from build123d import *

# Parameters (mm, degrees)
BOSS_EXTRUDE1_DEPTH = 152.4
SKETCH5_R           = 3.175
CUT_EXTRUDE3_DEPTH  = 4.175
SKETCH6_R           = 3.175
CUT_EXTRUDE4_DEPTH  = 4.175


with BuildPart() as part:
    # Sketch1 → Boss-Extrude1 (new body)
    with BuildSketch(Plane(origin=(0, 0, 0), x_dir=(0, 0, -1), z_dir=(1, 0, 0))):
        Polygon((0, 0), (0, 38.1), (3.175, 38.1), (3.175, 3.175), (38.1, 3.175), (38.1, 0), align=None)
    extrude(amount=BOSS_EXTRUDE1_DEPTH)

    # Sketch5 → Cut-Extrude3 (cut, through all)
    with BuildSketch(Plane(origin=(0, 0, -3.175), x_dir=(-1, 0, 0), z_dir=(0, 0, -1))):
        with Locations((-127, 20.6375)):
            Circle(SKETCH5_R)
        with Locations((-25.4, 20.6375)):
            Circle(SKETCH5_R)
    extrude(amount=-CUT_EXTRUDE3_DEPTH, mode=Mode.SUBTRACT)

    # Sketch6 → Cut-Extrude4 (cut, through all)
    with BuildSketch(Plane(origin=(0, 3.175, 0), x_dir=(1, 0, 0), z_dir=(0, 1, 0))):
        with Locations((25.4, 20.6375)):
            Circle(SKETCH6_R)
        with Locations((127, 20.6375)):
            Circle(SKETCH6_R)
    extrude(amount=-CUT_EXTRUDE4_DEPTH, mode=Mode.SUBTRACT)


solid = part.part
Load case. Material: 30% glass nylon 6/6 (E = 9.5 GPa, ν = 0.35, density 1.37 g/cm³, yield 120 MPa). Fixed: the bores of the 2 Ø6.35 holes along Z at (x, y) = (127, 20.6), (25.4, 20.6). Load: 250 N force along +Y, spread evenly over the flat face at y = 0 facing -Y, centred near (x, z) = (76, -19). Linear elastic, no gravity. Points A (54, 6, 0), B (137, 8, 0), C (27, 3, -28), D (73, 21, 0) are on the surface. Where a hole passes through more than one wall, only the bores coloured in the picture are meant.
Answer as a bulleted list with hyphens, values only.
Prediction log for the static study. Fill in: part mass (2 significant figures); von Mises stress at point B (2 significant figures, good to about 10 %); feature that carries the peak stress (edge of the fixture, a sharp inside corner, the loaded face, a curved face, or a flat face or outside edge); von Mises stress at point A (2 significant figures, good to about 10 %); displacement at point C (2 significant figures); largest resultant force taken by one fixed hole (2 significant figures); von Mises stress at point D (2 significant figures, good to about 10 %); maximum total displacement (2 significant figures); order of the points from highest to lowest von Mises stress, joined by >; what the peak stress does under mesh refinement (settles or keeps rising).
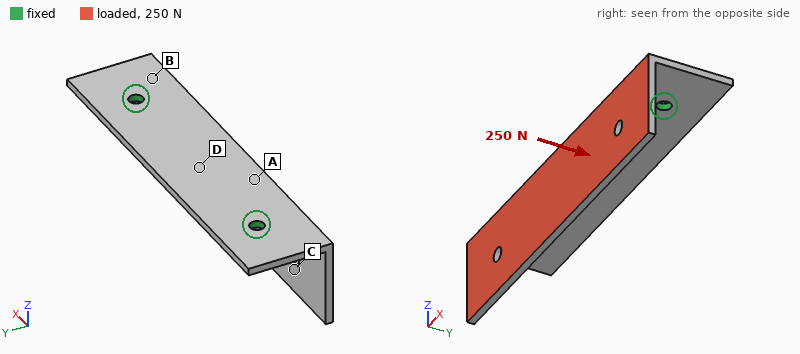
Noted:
- 48 g
- 18 MPa
- edge of the fixture
- 13 MPa
- 0.92 mm
- 130 N
- 6.1 MPa
- 1.4 mm
- B > A > D > C
- keeps rising
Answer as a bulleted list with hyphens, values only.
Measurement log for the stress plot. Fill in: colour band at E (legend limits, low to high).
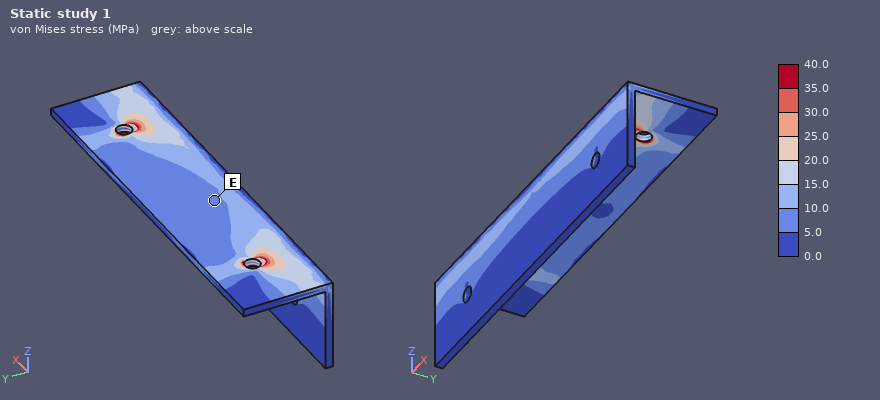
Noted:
- 5.0 to 10.0 MPa
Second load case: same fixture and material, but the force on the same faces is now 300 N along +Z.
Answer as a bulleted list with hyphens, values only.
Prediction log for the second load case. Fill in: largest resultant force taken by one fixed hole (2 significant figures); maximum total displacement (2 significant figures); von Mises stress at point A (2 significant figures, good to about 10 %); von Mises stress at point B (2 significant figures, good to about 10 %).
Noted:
- 150 N
- 0.97 mm
- 5.5 MPa
- 14 MPa
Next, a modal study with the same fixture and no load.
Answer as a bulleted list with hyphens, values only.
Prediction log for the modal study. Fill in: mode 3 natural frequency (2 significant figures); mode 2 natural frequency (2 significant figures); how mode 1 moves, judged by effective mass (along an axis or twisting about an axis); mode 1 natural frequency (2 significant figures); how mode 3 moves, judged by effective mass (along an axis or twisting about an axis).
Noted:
- 1100 Hz
- 710 Hz
- along Y
- 490 Hz
- along Z
